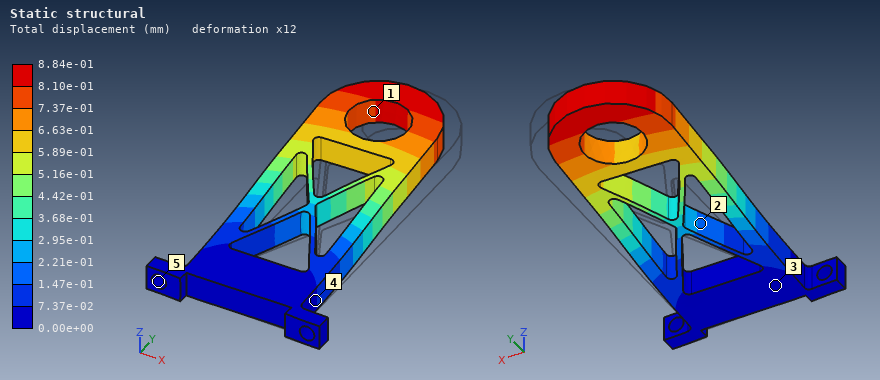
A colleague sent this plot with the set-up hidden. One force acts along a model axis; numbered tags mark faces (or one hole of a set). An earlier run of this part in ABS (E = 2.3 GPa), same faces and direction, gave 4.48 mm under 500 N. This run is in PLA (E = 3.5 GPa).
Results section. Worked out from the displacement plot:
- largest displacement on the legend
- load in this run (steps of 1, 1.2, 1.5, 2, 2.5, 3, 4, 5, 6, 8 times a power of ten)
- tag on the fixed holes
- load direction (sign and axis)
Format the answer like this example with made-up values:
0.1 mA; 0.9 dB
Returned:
8.84e-01 mm; 150 N; 5; -X
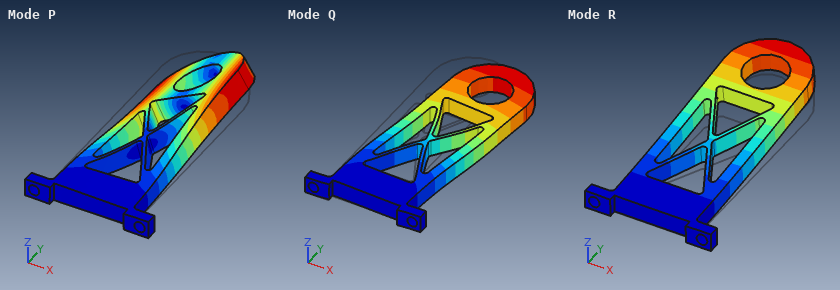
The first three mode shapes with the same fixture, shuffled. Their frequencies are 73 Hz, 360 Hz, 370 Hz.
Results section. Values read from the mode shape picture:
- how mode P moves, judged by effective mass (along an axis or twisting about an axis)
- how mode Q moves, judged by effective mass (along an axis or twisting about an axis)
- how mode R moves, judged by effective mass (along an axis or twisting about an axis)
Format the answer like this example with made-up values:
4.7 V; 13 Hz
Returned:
twisting about Y; along X; along Z
